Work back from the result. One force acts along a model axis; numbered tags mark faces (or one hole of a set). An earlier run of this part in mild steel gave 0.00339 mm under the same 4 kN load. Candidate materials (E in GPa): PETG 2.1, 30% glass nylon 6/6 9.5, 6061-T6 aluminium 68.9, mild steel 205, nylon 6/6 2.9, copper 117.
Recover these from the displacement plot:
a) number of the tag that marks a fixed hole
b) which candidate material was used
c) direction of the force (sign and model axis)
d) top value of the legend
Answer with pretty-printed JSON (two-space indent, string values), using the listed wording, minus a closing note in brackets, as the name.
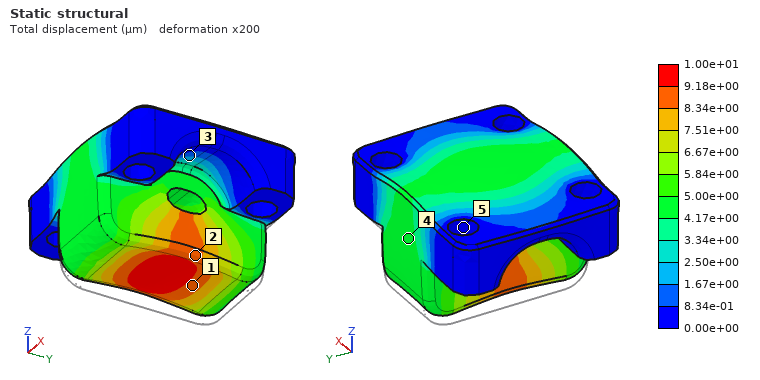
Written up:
{
  "number of the tag that marks a fixed hole": "5",
  "which candidate material was used": "6061-T6 aluminium",
  "direction of the force": "+Z",
  "top value of the legend": "1.00e+01 µm"
}
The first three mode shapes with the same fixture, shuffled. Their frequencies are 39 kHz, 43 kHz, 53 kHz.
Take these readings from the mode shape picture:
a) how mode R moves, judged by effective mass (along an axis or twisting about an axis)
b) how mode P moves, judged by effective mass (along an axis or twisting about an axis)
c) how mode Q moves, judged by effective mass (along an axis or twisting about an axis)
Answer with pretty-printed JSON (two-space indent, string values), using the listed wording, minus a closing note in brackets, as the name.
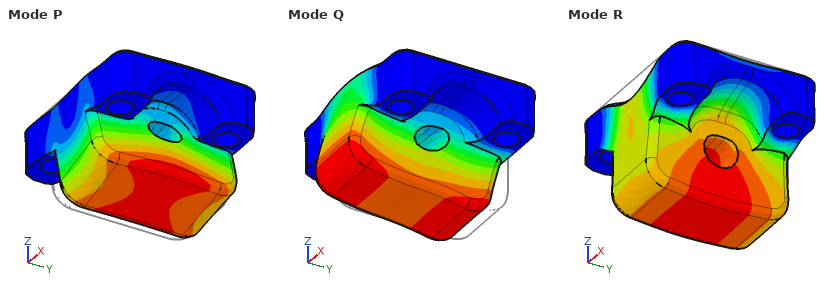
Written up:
{
  "how mode R moves, judged by effective mass": "along Z",
  "how mode P moves, judged by effective mass": "along X",
  "how mode Q moves, judged by effective mass": "along Y"
}
